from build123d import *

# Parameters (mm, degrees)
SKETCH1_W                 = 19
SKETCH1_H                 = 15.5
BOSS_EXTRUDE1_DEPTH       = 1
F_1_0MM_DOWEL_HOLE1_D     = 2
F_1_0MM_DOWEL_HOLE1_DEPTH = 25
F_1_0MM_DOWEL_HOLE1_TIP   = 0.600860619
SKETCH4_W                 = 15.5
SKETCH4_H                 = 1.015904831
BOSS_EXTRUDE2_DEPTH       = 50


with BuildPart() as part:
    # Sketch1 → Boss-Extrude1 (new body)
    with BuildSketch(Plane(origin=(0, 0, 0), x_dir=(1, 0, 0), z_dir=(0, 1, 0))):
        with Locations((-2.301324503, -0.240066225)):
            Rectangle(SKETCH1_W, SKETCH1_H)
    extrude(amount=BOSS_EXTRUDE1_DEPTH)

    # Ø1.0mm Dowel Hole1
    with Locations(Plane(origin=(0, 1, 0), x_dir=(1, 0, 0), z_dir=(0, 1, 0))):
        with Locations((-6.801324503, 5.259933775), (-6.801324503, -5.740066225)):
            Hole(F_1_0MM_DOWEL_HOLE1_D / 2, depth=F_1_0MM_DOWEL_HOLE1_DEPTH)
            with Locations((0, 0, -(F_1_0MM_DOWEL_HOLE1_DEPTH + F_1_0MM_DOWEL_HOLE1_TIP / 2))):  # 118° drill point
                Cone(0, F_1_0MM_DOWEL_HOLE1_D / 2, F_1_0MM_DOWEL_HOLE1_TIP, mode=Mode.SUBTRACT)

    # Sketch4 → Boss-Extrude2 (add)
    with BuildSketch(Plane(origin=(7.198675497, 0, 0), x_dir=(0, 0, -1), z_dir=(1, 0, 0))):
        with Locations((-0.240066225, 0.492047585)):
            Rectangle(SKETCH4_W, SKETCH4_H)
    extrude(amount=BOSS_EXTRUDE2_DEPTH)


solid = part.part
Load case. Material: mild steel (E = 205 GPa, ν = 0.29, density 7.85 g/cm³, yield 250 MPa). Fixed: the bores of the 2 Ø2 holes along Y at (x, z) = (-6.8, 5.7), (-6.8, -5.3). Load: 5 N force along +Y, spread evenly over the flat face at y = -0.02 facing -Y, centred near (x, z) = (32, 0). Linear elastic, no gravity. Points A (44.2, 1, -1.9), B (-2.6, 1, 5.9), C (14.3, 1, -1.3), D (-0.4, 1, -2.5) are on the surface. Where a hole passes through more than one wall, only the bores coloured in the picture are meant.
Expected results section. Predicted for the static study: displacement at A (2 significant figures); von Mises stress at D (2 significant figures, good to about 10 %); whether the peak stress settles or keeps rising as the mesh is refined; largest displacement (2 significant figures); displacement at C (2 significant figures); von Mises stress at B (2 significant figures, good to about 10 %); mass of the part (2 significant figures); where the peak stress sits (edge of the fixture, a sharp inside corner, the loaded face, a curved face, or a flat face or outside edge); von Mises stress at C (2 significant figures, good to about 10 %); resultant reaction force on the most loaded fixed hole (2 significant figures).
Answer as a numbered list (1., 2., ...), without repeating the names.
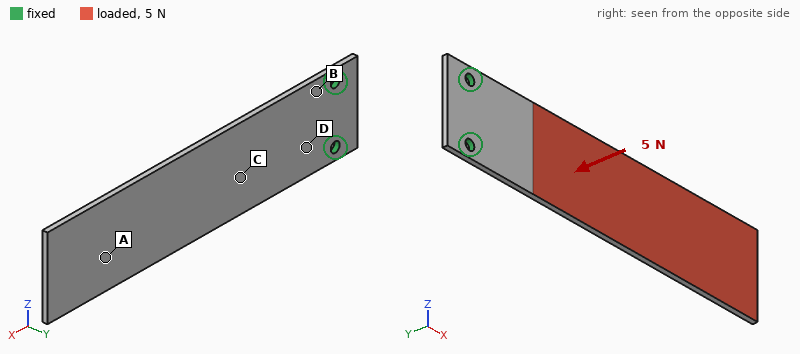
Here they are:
1. 0.55 mm
2. 59 MPa
3. keeps rising
4. 0.75 mm
5. 0.13 mm
6. 66 MPa
7. 8.4 g
8. edge of the fixture
9. 34 MPa
10. 2.5 N
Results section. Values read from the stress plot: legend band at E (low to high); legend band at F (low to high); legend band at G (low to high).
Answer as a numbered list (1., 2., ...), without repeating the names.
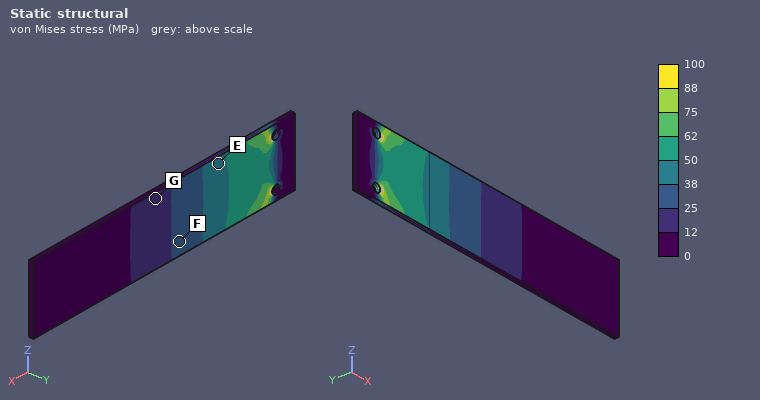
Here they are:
1. 38 to 50 MPa
2. 25 to 38 MPa
3. 12 to 25 MPa
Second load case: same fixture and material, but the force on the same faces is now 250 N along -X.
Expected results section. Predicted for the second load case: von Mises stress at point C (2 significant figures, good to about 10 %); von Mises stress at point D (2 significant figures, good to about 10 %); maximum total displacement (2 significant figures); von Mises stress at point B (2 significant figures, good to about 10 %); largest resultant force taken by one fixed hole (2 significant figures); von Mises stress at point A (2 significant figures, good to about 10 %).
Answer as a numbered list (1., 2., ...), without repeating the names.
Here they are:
1. 27 MPa
2. 32 MPa
3. 0.75 mm
4. 30 MPa
5. 130 N
6. 8.4 MPa
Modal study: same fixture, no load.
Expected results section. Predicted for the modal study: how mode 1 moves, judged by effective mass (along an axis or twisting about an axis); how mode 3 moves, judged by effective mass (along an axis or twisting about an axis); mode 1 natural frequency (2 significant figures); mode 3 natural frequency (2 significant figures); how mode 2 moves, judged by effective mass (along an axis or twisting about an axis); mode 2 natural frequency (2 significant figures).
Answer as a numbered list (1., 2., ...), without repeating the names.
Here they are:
1. along Y
2. twisting about X
3. 200 Hz
4. 1700 Hz
5. along Y
6. 1300 Hz
